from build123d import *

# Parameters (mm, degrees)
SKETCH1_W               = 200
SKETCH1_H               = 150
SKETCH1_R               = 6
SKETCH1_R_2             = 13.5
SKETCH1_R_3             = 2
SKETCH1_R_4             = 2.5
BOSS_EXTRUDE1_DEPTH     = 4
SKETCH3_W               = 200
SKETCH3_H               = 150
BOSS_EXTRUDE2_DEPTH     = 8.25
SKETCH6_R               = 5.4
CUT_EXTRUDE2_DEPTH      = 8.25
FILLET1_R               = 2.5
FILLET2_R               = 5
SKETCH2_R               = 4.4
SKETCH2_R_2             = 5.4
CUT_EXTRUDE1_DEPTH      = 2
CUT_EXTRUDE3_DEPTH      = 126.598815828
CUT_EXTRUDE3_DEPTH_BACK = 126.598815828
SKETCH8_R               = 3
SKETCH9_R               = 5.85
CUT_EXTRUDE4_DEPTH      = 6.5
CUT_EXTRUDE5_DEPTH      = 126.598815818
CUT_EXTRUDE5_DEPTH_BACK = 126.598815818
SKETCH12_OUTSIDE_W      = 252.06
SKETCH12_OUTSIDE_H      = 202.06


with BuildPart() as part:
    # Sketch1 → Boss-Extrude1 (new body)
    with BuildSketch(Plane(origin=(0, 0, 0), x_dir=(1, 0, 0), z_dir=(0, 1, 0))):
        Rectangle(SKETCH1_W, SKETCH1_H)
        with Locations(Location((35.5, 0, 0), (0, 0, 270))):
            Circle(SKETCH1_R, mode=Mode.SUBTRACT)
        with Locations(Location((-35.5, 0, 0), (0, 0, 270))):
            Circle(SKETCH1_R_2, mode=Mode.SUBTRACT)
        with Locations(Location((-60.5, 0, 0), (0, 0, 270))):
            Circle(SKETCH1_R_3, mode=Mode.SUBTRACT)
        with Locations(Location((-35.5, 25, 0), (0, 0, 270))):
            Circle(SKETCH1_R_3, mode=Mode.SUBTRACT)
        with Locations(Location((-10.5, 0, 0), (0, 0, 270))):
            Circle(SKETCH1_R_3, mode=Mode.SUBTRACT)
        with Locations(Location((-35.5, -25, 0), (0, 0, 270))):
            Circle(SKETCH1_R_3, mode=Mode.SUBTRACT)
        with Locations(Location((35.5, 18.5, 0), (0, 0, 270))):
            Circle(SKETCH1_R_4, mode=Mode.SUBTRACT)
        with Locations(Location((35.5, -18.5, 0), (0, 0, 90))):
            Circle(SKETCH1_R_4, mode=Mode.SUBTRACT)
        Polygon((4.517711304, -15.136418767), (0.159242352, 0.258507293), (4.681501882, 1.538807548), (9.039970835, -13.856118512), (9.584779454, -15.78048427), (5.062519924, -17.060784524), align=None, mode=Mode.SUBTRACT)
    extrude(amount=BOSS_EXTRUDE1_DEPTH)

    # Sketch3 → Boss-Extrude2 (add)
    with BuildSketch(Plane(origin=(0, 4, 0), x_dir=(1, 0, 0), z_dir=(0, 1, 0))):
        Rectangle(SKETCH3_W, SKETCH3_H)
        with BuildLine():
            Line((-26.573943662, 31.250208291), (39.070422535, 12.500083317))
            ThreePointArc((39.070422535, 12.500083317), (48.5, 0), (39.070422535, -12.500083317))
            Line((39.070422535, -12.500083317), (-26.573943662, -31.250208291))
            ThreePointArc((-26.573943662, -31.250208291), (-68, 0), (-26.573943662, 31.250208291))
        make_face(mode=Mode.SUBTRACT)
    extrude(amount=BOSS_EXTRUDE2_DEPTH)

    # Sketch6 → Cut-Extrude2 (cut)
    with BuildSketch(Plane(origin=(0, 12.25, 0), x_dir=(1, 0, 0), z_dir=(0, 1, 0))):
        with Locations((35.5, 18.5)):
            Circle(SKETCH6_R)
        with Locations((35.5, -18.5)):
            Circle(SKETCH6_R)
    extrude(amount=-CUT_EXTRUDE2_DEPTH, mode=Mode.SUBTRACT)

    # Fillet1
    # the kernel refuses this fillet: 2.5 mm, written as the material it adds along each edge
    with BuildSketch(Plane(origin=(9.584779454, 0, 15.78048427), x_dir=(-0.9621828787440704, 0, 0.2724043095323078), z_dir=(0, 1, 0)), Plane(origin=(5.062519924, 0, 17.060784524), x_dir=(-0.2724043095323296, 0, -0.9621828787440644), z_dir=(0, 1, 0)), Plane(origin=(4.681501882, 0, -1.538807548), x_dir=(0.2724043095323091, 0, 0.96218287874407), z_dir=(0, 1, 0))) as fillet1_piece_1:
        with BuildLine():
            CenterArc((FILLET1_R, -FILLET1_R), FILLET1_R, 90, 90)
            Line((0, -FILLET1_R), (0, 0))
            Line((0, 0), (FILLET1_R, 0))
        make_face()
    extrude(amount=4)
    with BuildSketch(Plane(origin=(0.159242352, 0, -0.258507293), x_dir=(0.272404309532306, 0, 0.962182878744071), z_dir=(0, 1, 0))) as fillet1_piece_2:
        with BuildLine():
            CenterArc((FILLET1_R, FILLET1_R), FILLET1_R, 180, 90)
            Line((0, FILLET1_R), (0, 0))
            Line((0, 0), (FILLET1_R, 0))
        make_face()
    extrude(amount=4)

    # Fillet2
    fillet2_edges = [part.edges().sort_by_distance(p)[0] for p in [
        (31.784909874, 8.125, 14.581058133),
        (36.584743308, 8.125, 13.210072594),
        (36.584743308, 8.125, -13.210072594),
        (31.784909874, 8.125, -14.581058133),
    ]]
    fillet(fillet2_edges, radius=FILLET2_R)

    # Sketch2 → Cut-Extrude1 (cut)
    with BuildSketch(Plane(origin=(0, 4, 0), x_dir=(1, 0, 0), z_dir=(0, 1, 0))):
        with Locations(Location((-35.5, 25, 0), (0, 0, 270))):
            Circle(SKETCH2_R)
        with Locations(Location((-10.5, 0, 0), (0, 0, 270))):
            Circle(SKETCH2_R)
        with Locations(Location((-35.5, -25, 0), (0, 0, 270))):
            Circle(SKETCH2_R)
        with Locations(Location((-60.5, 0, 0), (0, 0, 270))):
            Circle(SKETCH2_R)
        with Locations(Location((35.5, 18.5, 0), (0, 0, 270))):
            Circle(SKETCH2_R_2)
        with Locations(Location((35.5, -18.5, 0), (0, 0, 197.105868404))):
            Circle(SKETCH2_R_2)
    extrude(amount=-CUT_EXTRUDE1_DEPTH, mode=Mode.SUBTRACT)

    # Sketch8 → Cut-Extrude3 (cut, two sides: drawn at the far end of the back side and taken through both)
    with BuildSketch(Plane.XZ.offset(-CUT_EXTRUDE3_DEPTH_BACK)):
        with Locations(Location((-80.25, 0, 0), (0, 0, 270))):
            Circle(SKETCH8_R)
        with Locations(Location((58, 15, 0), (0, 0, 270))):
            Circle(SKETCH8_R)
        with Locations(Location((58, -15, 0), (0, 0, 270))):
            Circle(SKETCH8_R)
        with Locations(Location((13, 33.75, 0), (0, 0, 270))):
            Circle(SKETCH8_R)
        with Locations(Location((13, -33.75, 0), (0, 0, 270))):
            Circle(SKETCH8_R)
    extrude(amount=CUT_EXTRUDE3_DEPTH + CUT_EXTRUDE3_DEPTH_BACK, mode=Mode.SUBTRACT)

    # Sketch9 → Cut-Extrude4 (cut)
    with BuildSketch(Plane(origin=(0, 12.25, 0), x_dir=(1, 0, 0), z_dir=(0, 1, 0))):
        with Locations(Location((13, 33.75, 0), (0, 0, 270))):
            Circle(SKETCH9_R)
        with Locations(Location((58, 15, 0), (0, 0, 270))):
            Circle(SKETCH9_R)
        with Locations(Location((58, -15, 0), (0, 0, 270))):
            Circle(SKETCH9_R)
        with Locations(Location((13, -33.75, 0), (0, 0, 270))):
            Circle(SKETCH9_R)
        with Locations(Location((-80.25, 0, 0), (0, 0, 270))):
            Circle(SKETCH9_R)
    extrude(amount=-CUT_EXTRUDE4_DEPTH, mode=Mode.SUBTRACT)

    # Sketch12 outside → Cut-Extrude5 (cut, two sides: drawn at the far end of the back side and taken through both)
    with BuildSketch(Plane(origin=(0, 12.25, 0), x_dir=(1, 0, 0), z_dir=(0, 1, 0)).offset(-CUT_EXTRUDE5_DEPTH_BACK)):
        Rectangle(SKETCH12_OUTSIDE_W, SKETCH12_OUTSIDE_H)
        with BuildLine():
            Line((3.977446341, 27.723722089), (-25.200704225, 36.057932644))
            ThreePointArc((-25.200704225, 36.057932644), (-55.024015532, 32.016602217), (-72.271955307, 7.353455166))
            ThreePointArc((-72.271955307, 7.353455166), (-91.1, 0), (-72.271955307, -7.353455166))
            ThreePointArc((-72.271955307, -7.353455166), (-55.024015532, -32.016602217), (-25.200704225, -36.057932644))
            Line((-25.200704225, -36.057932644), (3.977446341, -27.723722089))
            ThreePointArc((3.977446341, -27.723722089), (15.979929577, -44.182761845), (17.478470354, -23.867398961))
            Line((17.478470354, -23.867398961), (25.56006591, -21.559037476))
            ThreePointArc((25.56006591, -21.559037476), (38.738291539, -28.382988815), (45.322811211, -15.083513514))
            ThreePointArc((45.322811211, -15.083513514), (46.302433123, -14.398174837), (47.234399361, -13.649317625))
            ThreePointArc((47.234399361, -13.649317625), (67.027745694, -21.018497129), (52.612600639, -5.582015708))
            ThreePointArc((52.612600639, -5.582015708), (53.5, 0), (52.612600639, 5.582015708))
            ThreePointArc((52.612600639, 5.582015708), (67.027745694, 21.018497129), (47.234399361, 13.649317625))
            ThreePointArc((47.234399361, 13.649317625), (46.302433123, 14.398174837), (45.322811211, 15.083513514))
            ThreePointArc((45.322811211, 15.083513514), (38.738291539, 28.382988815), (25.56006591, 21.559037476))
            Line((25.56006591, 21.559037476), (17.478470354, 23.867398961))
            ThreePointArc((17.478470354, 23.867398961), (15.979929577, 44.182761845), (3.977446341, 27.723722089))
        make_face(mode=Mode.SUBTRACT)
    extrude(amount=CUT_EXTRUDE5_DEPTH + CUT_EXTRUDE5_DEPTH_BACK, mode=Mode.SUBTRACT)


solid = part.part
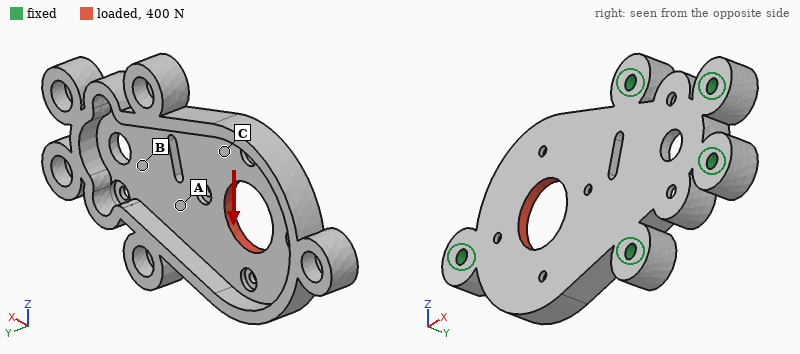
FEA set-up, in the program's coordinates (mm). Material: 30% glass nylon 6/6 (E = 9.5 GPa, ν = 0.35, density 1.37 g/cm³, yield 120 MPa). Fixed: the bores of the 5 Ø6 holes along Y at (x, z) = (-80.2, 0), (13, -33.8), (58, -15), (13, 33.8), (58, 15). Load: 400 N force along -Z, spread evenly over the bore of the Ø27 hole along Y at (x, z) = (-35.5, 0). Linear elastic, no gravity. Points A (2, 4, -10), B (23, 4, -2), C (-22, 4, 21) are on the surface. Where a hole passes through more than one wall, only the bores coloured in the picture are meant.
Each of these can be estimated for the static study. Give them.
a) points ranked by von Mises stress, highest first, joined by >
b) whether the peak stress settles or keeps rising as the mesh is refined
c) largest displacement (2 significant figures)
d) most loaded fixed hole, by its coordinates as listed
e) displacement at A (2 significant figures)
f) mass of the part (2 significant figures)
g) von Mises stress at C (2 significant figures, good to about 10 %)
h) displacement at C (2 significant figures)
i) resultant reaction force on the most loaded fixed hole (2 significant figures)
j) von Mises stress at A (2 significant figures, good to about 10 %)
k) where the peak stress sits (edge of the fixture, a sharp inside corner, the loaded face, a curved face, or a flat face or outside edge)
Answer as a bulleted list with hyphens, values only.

- A > C > B
- keeps rising
- 19 µm
- (-80.2, 0)
- 4.6 µm
- 76 g
- 0.96 MPa
- 12 µm
- 180 N
- 2.0 MPa
- edge of the fixture
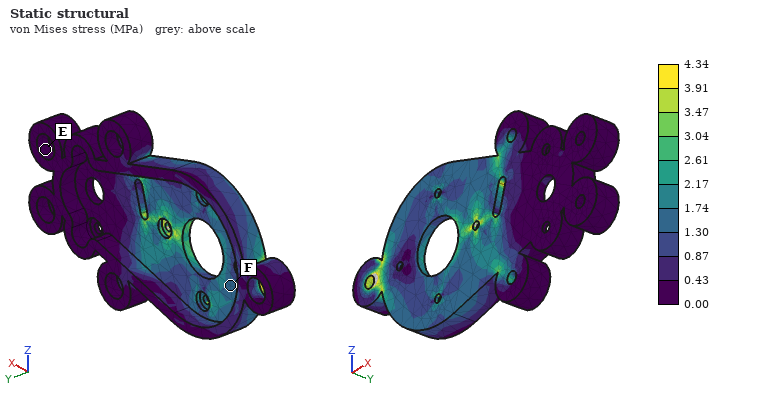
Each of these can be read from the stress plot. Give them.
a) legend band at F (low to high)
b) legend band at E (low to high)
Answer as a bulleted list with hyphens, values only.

- 1.30 to 1.74 MPa
- 0.00 to 0.43 MPa
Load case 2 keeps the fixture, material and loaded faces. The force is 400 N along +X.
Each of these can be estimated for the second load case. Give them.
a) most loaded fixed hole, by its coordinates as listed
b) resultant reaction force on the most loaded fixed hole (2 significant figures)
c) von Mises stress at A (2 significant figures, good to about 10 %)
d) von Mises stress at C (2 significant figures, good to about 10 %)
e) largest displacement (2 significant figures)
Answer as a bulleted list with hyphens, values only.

- (-80.2, 0)
- 170 N
- 0.72 MPa
- 0.86 MPa
- 7.9 µm
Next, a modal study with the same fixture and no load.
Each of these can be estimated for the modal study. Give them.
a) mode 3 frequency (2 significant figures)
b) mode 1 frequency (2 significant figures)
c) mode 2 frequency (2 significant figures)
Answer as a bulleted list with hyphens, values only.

- 2900 Hz
- 1800 Hz
- 1900 Hz
